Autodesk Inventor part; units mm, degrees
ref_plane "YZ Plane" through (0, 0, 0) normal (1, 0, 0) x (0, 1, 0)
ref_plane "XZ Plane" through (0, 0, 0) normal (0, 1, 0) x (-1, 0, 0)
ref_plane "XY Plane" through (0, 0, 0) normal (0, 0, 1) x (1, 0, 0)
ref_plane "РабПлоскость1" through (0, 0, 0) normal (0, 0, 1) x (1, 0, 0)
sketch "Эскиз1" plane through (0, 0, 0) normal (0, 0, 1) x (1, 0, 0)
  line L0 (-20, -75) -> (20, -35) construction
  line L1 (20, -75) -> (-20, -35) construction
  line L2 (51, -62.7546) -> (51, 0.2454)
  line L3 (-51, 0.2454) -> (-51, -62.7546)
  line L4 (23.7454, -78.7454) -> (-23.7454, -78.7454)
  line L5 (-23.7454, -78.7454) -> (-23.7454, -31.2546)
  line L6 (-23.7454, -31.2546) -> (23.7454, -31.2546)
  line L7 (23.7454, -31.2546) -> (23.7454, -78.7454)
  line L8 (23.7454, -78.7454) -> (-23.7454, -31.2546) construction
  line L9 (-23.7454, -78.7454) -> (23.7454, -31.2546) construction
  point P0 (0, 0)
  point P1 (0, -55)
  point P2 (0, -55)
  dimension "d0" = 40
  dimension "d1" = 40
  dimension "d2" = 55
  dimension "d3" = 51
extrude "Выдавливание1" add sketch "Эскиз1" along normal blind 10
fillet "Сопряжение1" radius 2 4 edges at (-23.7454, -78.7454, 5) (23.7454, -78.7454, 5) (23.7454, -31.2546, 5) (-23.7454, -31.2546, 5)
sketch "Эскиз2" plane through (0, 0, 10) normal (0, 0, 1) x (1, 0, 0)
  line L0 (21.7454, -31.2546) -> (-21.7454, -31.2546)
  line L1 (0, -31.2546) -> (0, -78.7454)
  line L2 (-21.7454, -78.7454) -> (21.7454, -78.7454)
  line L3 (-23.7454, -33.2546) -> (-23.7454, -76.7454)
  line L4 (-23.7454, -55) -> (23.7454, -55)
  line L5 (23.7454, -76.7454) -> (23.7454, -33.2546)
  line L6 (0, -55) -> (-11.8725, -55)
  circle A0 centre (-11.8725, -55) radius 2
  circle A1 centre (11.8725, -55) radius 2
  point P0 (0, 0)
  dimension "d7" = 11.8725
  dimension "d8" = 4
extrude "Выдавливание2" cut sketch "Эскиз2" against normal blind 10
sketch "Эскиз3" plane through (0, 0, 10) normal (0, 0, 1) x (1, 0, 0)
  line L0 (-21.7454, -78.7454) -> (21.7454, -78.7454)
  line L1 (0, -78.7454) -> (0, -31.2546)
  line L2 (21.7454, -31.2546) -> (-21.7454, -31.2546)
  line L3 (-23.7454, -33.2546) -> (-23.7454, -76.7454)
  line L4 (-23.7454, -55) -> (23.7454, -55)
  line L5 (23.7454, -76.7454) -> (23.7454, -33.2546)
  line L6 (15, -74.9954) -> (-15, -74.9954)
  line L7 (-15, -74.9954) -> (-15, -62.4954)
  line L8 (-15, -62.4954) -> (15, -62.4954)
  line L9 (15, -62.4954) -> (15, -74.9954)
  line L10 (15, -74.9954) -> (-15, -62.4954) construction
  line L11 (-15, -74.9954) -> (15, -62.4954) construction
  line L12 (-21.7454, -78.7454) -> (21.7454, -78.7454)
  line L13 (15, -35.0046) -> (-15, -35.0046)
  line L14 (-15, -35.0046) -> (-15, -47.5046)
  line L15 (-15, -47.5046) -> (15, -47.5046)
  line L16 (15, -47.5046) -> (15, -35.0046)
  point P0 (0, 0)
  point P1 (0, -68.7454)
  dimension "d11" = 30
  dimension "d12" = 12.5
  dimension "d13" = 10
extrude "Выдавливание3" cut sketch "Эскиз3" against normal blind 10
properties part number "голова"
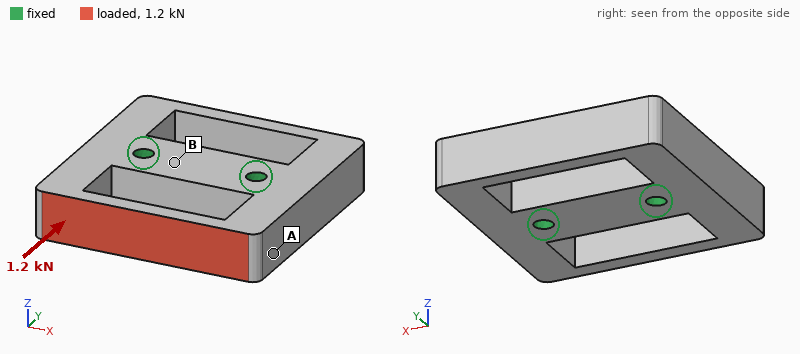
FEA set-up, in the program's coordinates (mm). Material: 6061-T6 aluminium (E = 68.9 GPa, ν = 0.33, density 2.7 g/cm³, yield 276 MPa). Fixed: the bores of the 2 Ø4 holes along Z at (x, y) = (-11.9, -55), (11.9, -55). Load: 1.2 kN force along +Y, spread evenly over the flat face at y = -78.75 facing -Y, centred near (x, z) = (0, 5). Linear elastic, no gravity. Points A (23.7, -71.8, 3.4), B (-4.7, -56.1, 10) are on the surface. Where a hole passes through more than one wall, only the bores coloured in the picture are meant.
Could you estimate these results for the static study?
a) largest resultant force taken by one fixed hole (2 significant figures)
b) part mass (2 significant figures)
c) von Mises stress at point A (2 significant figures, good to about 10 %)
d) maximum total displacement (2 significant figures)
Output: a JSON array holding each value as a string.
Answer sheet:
["620 N", "40 g", "14 MPa", "43 µm"]
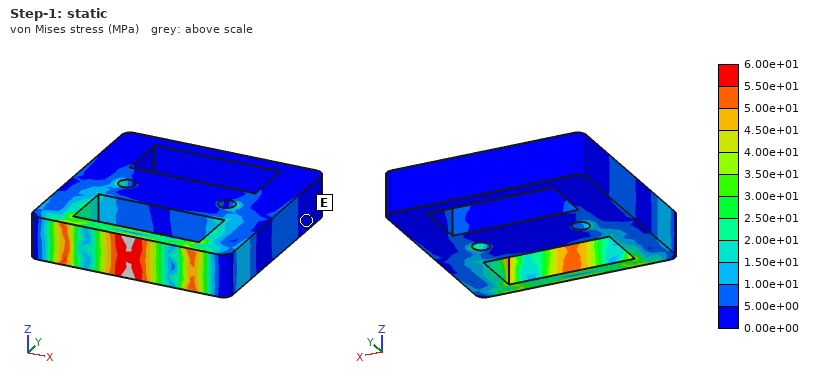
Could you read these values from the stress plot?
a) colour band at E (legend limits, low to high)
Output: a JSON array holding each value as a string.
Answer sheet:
["0.00e+00 to 5.00e+00 MPa"]
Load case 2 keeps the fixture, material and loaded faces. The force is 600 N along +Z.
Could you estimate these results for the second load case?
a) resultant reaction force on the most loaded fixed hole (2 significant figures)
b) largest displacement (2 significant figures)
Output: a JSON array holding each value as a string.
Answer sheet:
["300 N", "46 µm"]
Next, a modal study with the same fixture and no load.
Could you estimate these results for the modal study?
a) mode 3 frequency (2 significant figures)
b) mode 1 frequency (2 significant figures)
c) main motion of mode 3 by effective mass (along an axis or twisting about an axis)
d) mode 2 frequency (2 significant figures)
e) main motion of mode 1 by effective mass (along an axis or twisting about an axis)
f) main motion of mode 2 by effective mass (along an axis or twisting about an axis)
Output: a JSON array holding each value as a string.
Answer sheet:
["10000 Hz", "7900 Hz", "along Z", "8700 Hz", "twisting about X", "twisting about Z"]
